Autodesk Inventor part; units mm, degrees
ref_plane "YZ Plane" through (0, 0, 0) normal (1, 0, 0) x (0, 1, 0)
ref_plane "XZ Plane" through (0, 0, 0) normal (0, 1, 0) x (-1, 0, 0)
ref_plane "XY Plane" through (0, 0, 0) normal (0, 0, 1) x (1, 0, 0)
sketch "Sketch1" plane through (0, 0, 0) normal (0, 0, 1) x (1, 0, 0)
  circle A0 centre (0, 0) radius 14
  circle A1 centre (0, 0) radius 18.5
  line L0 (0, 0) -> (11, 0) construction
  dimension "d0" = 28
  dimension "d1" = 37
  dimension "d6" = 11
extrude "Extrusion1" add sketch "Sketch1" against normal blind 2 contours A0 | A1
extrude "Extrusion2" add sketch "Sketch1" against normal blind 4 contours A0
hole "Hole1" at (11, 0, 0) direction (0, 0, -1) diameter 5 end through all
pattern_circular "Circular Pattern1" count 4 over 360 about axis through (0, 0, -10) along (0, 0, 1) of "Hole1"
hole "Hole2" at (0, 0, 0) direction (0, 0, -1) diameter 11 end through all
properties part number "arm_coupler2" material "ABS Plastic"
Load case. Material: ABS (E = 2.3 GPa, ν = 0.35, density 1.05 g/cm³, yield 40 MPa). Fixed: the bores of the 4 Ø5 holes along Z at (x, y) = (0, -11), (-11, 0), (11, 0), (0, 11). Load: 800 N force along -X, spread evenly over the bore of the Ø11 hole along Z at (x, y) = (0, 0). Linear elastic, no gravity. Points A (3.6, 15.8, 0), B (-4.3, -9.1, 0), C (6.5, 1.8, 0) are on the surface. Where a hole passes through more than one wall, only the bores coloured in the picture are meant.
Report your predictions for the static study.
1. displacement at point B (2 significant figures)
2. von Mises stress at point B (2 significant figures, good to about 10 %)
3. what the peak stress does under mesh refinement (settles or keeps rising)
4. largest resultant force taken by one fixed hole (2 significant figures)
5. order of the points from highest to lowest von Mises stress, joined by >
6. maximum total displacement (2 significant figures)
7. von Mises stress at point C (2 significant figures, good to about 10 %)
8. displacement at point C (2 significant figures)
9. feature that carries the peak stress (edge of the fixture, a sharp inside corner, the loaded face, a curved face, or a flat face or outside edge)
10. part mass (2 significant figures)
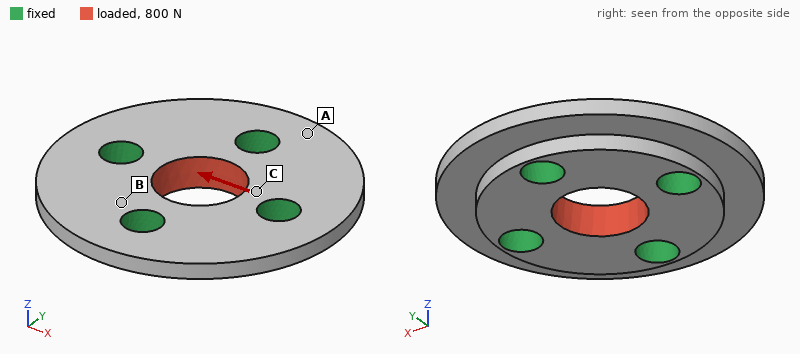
6.0 µm
3.1 MPa
keeps rising
240 N
C > B > A
20 µm
7.4 MPa
9.0 µm
edge of the fixture
2.8 g
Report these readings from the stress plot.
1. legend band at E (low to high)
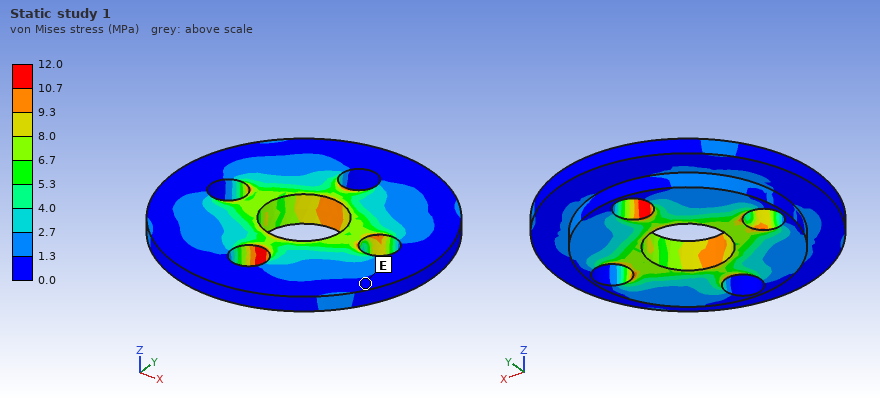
0.0 to 1.3 MPa
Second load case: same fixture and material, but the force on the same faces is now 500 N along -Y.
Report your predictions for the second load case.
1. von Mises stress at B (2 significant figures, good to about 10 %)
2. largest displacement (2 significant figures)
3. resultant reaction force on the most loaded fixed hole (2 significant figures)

2.1 MPa
13 µm
150 N
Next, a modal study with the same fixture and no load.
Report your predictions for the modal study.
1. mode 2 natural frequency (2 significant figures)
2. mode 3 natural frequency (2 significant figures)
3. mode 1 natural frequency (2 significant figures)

11 kHz
11 kHz
11 kHz
